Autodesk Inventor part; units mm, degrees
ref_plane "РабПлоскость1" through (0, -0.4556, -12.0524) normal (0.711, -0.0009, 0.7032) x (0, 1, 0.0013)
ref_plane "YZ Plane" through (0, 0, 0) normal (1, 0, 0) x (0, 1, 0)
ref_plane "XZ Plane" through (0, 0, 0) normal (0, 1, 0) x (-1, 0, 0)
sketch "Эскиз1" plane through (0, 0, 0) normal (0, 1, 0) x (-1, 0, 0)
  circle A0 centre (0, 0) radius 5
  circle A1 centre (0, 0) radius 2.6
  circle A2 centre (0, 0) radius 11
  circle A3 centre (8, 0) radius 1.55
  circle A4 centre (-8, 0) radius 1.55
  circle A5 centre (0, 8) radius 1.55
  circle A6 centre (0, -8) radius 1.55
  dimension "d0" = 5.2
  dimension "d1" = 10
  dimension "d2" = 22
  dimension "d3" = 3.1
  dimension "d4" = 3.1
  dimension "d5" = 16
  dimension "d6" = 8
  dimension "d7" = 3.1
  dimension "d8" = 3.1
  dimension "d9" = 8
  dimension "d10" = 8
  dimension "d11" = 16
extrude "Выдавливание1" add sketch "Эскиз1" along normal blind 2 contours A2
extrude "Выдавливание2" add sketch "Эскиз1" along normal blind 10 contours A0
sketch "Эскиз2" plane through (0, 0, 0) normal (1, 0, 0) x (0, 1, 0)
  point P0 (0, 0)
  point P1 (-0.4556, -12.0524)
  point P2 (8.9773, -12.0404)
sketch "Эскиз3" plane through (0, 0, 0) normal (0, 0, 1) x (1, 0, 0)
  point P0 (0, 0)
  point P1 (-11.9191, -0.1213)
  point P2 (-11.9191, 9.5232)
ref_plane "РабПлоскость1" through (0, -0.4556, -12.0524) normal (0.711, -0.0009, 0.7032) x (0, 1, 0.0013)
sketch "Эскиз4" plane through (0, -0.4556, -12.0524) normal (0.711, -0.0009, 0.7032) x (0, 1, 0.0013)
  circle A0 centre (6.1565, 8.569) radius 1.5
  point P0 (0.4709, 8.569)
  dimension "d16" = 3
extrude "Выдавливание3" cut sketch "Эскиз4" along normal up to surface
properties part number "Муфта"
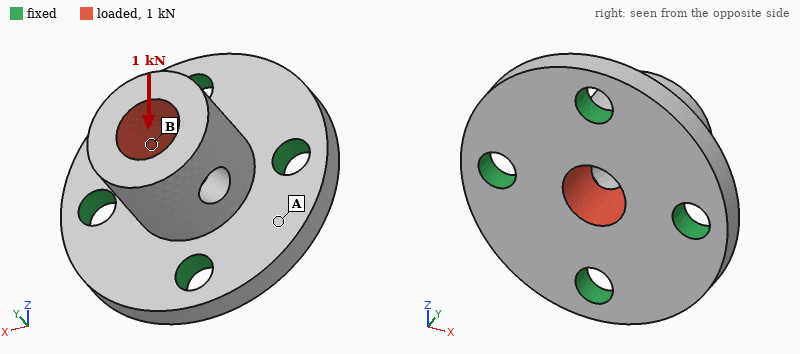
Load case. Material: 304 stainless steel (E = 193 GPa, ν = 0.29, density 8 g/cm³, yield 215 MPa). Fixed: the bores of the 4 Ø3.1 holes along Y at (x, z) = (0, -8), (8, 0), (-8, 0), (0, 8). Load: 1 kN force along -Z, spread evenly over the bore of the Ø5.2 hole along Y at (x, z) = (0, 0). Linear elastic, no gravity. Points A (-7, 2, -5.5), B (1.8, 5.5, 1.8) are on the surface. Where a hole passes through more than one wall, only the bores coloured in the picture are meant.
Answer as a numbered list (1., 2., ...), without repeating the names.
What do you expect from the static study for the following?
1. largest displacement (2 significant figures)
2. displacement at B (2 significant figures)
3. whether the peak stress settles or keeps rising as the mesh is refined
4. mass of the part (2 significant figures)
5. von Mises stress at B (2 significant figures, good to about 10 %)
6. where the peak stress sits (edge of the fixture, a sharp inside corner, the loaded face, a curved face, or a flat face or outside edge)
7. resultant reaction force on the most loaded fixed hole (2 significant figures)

1. 5.4 µm
2. 2.6 µm
3. keeps rising
4. 8.8 g
5. 31 MPa
6. edge of the fixture
7. 460 N
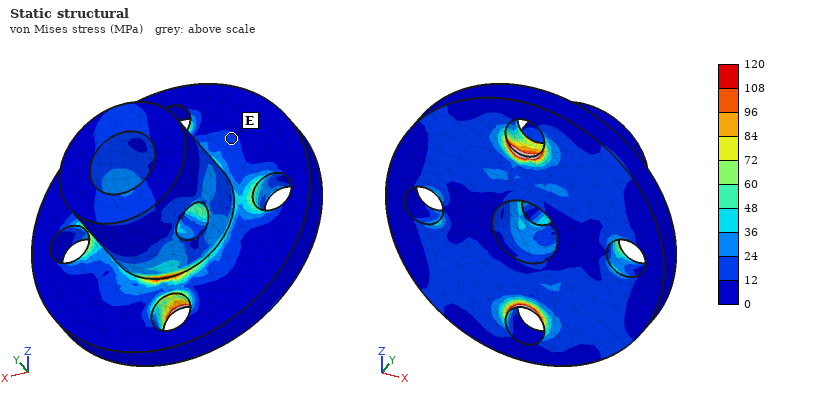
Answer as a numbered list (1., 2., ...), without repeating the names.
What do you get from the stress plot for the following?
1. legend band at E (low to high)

1. 12 to 24 MPa
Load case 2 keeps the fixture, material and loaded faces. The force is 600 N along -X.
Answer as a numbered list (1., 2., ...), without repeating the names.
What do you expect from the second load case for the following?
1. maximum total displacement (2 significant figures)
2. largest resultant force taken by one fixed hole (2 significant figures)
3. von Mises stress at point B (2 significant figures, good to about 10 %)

1. 3.2 µm
2. 270 N
3. 18 MPa
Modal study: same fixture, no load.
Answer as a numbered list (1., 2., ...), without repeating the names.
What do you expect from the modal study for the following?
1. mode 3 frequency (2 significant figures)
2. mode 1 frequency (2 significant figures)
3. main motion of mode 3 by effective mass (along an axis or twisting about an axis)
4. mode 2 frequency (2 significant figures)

1. 55 kHz
2. 37 kHz
3. along Y
4. 38 kHz
